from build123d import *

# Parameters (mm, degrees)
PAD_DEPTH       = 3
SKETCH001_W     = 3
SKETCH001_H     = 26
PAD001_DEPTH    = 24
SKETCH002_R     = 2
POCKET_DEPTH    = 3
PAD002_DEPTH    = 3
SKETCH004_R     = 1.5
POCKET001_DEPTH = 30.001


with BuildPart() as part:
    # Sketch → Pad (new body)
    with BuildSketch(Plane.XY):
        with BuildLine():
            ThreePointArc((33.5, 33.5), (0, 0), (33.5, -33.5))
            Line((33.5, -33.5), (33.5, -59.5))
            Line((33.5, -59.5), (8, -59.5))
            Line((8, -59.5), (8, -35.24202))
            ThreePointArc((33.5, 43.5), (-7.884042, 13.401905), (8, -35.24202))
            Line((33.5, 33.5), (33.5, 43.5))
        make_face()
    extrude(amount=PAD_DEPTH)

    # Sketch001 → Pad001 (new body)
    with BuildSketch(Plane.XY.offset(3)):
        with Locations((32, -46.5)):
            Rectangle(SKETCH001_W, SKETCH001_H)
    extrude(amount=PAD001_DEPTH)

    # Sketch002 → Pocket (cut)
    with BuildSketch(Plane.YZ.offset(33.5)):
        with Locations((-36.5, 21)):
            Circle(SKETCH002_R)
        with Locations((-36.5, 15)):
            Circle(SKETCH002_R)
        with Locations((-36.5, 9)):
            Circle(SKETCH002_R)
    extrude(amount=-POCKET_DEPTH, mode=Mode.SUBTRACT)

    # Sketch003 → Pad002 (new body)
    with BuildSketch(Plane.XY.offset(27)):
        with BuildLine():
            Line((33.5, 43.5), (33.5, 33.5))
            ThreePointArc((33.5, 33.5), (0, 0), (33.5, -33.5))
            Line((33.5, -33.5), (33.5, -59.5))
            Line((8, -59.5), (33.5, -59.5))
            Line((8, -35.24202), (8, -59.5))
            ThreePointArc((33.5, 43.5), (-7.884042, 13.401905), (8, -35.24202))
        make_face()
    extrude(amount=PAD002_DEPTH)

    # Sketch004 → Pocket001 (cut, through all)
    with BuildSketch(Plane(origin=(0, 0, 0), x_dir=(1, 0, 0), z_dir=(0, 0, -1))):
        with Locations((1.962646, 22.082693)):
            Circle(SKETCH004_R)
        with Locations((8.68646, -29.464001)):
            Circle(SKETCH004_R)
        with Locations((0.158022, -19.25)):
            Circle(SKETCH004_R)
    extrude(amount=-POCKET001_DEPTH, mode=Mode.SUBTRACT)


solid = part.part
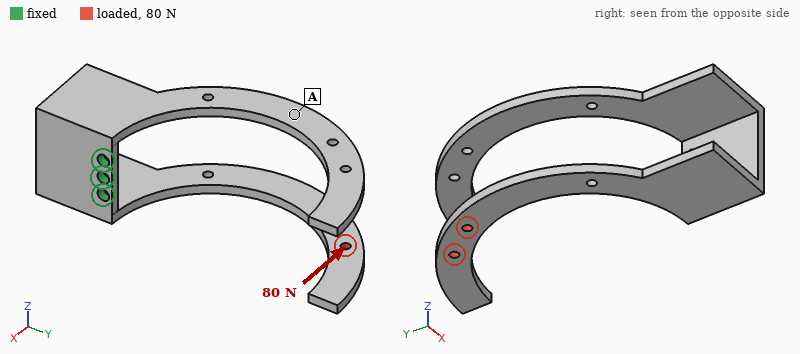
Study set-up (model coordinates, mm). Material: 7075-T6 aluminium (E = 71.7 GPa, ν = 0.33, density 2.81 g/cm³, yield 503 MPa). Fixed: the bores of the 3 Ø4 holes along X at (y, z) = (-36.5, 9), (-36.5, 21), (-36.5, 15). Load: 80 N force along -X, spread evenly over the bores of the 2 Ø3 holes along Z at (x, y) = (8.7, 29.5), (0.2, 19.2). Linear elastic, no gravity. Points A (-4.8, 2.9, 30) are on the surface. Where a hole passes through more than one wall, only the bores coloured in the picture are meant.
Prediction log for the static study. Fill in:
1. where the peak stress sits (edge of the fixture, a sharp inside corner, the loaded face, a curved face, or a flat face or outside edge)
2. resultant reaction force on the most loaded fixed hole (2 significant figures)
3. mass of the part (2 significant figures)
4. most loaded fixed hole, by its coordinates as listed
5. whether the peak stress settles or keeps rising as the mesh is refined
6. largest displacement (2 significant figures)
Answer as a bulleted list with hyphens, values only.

- edge of the fixture
- 100 N
- 33 g
- (-36.5, 9)
- keeps rising
- 1.2 mm
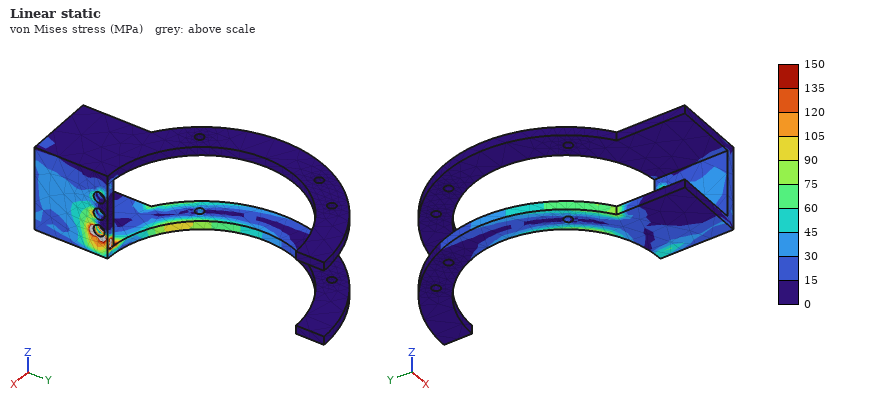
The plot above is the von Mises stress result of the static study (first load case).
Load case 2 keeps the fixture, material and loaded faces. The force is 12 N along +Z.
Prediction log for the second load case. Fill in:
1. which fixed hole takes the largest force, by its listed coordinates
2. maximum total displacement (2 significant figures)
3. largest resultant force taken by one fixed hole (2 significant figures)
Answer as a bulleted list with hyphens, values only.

- (-36.5, 9)
- 1.2 mm
- 57 N
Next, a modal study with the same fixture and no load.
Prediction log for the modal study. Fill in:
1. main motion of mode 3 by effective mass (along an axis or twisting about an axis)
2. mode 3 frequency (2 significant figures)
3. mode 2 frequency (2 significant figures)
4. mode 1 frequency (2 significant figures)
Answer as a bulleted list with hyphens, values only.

- along X
- 590 Hz
- 250 Hz
- 250 Hz
